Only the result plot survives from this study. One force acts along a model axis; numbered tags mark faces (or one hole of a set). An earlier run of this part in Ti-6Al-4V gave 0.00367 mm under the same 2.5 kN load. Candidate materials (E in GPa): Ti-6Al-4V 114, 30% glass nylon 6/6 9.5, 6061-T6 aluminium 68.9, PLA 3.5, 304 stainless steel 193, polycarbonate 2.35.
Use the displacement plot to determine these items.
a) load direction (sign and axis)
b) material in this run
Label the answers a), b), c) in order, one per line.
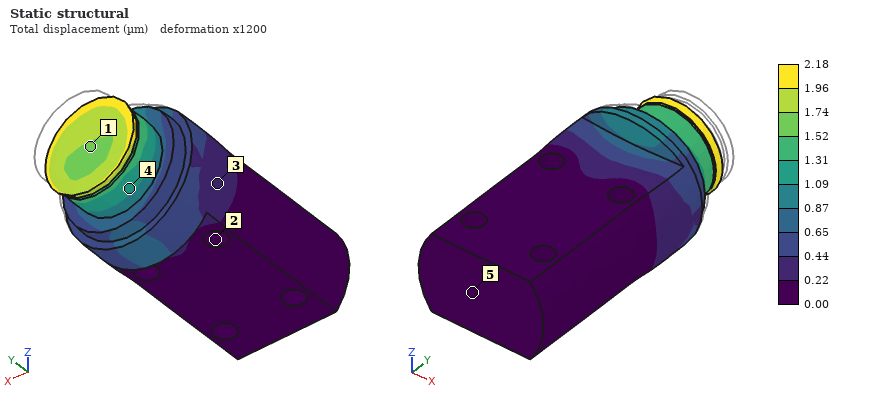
a) -Y
b) 304 stainless steel
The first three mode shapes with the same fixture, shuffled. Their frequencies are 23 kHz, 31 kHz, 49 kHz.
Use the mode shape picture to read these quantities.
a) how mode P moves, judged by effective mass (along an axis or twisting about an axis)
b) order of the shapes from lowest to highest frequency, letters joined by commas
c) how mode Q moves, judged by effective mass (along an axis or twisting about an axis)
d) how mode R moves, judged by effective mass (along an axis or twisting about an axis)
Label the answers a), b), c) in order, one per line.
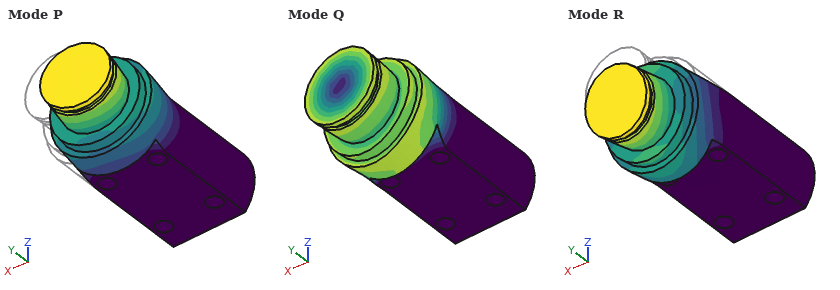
a) along X
b) R, P, Q
c) twisting about Y
d) along Z
